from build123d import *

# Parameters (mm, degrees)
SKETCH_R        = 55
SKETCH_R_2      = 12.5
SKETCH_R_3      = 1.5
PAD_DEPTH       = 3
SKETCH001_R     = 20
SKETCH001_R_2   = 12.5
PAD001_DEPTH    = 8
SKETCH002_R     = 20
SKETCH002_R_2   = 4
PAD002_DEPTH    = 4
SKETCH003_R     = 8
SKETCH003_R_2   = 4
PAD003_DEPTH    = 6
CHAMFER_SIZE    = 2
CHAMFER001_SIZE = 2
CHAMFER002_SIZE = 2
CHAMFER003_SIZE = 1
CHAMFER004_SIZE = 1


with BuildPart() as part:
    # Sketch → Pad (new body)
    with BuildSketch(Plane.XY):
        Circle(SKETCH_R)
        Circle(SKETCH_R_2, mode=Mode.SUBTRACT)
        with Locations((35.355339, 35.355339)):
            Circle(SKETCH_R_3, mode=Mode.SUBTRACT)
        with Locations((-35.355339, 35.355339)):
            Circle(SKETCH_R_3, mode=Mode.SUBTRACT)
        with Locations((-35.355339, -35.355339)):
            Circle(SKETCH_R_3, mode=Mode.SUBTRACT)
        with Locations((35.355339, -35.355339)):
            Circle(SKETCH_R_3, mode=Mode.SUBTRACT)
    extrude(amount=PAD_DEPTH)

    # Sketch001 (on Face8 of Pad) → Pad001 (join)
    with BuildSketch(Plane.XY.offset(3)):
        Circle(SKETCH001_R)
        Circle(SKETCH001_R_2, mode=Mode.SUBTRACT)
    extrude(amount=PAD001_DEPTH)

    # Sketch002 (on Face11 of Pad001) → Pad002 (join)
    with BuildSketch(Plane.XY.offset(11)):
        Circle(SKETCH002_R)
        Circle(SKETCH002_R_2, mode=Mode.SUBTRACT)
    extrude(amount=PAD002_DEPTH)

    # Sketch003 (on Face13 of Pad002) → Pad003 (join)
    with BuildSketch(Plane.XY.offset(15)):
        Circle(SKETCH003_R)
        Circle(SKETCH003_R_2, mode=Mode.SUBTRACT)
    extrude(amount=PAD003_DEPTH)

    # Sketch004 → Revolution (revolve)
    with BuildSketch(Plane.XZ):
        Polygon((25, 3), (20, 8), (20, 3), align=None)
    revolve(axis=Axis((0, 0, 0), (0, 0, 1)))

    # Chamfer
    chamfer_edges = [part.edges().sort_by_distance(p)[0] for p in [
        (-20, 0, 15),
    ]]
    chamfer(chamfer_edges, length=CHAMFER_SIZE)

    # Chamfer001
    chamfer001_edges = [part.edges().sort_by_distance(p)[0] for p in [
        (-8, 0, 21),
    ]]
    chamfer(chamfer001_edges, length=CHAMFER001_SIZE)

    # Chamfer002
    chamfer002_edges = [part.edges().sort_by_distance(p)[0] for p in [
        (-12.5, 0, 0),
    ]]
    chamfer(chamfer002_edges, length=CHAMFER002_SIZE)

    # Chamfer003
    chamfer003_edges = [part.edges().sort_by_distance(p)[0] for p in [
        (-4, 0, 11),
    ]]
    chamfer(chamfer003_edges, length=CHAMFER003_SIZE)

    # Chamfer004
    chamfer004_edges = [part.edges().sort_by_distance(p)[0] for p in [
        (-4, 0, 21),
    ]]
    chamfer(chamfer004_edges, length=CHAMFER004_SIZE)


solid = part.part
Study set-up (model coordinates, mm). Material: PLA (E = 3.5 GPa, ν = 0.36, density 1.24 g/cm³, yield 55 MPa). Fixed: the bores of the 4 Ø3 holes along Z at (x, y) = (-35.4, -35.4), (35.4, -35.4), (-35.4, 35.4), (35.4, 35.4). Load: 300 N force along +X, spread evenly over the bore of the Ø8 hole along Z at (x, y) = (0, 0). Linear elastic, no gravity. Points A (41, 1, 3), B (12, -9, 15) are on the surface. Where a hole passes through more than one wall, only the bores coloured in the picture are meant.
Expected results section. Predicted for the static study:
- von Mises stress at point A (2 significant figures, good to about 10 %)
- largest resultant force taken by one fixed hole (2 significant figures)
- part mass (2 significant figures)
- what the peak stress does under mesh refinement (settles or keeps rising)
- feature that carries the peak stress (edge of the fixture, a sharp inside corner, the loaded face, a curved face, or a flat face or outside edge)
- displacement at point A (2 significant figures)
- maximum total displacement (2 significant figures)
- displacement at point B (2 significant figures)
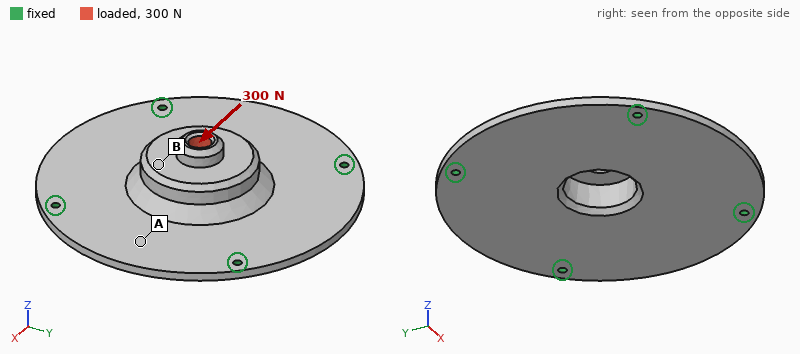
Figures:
2.9 MPa
86 N
50 g
keeps rising
edge of the fixture
0.24 mm
0.25 mm
0.18 mm
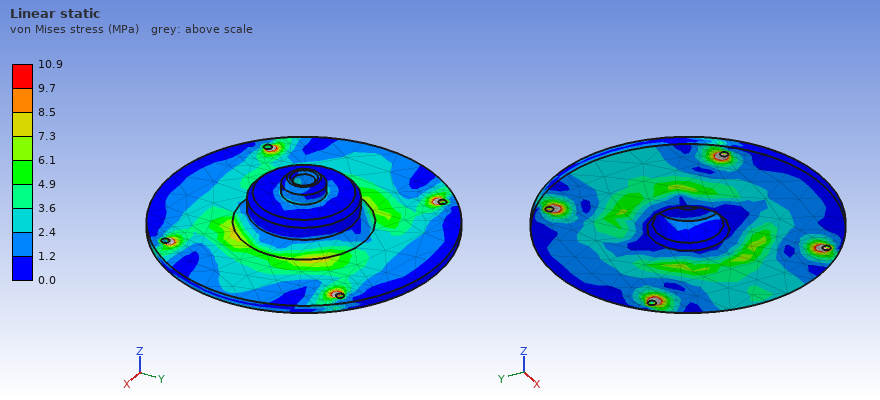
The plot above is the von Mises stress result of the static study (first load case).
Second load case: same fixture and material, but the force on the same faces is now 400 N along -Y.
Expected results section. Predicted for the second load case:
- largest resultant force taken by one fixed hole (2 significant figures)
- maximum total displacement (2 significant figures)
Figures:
110 N
0.33 mm
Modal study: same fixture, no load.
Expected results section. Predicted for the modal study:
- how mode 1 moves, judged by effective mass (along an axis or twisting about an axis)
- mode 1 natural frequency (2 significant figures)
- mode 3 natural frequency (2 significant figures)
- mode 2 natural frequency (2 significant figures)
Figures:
along Z
660 Hz
910 Hz
910 Hz
